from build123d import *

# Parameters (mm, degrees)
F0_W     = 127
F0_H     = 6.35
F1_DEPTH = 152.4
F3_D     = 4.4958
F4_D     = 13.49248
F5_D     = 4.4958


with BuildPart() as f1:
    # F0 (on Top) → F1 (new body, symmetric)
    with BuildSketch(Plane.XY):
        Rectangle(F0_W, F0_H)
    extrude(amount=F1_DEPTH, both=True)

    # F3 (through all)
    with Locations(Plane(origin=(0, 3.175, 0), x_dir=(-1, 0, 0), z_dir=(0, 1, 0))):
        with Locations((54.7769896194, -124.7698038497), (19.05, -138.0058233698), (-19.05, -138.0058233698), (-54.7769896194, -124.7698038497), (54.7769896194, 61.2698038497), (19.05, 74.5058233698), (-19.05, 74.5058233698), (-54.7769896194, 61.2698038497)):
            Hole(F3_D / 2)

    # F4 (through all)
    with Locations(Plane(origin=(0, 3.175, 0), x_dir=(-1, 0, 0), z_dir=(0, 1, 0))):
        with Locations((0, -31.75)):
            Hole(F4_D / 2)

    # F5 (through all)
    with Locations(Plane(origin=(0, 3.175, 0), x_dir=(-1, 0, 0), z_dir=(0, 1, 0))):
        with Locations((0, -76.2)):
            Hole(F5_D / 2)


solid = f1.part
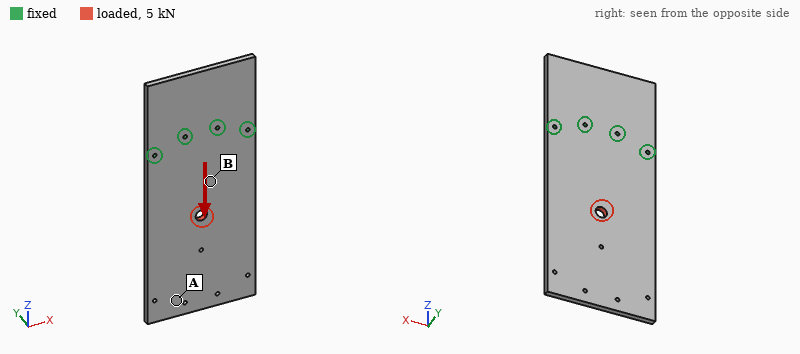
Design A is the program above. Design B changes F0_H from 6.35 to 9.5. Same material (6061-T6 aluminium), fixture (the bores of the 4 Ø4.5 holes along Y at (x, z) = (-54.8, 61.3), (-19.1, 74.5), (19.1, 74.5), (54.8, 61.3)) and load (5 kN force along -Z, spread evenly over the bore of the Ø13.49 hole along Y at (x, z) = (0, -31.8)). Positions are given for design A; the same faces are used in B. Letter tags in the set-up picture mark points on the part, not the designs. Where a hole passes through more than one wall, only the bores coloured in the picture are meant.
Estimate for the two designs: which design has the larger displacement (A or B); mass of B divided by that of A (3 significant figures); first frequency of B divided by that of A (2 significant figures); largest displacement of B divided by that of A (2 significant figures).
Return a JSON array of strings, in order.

["A", "1.50", "1.5", "0.67"]
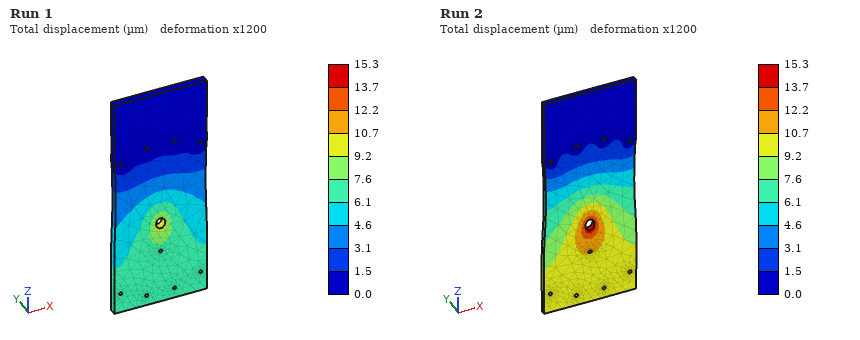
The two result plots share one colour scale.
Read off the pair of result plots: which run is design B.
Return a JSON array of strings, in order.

["Run 1"]
